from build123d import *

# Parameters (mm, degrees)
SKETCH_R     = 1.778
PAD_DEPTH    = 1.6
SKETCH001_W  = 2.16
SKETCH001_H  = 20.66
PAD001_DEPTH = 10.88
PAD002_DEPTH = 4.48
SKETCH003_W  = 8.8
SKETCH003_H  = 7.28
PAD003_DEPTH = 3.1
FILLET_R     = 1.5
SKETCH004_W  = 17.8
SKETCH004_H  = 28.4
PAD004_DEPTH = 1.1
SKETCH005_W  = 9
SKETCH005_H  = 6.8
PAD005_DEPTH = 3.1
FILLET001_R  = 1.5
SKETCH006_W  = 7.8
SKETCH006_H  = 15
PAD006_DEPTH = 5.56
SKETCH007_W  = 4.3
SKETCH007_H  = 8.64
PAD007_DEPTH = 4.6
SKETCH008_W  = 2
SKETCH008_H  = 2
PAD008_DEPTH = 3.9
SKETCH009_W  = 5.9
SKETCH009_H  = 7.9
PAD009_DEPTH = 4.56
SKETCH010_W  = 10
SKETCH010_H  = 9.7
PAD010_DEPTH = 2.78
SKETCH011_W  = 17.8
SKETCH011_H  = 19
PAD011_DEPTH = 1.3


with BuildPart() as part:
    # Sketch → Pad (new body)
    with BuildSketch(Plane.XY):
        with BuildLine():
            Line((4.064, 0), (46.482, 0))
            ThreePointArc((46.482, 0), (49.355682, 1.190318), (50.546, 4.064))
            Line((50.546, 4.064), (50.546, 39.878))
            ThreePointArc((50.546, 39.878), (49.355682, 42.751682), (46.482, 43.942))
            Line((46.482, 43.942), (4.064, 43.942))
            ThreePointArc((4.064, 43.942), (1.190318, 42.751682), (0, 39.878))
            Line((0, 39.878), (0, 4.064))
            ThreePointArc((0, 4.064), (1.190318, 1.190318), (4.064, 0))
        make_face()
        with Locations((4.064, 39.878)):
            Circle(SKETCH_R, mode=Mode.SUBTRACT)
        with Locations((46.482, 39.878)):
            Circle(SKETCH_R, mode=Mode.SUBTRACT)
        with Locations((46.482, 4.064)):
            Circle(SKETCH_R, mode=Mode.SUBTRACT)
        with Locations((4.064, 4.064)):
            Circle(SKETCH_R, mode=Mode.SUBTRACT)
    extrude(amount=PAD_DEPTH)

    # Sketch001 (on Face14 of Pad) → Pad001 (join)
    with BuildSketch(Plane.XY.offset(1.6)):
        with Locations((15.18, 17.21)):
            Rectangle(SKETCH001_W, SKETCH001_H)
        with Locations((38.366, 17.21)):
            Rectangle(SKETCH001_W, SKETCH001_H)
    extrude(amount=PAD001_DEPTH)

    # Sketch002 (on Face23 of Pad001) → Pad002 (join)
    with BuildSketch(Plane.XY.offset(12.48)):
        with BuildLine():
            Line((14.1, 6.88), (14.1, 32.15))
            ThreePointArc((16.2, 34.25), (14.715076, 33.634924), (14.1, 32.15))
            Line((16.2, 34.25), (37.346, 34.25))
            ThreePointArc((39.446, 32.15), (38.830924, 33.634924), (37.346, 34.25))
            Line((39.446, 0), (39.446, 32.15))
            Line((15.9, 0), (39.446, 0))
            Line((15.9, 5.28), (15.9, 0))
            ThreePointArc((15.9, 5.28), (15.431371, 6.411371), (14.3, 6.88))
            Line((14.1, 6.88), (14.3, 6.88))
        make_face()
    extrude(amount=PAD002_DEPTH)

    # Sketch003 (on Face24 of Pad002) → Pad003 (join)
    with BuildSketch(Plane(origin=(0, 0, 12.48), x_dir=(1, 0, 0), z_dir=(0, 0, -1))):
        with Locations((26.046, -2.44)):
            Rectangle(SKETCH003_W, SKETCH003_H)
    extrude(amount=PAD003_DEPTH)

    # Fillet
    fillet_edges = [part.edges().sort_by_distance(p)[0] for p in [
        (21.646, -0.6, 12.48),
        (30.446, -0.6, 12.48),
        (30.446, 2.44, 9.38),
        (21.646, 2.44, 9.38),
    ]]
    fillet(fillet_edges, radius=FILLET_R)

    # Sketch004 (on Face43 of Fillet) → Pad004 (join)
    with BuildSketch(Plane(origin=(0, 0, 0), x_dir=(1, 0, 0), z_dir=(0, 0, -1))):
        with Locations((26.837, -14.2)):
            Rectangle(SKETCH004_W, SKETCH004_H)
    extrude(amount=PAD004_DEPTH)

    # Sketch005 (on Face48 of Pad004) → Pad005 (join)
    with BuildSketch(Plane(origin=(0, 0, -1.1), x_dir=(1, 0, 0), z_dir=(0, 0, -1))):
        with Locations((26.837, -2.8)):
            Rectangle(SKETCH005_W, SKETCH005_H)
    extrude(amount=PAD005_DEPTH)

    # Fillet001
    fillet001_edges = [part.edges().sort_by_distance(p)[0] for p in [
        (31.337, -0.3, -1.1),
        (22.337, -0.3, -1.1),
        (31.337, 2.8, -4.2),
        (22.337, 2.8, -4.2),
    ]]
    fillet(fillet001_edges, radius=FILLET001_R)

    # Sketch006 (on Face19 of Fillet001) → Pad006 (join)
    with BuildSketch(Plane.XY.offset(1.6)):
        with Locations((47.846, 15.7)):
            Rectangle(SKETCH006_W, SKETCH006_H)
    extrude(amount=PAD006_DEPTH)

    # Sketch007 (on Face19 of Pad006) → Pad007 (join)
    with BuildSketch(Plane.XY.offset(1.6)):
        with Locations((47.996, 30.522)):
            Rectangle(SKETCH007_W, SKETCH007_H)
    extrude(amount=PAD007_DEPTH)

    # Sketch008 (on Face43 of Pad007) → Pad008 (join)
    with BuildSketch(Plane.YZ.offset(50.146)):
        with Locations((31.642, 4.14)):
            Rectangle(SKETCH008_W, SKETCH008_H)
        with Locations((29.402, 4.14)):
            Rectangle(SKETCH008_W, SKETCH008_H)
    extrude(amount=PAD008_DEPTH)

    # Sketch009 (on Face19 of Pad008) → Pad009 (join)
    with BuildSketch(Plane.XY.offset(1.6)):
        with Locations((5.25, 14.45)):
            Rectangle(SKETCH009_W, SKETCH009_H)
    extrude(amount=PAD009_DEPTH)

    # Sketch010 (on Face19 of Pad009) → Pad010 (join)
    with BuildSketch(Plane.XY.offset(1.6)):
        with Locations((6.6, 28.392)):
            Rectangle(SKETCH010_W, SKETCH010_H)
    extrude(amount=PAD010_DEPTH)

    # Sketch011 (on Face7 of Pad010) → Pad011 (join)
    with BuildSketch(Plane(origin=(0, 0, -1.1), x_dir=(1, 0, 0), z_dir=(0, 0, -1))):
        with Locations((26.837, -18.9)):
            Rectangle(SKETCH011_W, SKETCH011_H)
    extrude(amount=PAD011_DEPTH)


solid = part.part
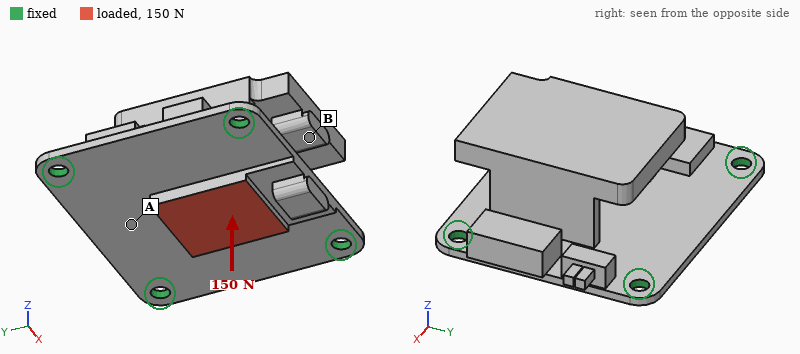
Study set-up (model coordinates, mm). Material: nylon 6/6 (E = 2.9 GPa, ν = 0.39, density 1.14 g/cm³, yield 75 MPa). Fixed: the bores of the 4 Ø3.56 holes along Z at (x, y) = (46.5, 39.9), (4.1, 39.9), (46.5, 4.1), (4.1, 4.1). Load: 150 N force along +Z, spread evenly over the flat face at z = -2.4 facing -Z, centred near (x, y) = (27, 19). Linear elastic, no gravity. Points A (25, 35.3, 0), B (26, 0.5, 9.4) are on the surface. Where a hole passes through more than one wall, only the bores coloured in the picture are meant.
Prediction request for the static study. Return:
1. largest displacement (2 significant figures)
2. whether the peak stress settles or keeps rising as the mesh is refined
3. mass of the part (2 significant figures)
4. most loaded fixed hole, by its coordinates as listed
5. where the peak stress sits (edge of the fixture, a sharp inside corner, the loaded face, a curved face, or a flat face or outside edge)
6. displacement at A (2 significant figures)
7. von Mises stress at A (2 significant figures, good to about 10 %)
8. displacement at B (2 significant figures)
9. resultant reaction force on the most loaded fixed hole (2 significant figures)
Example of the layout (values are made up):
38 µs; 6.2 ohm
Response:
0.66 mm; keeps rising; 13 g; (46.5, 4.1); edge of the fixture; 0.54 mm; 8.2 MPa; 0.23 mm; 53 N
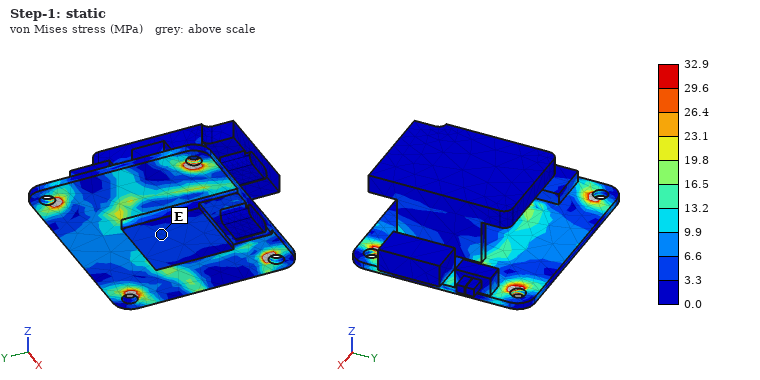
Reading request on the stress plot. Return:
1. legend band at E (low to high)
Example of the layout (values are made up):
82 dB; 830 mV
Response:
3.3 to 6.6 MPa
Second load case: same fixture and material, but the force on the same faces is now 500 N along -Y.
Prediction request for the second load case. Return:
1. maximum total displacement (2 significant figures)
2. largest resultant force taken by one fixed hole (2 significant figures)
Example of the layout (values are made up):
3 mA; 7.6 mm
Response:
0.53 mm; 170 N
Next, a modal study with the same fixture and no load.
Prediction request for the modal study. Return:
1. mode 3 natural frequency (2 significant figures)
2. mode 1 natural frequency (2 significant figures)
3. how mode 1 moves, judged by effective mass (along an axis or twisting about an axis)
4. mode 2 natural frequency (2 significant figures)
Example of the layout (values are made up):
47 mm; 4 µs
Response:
1300 Hz; 900 Hz; along Z; 1100 Hz
